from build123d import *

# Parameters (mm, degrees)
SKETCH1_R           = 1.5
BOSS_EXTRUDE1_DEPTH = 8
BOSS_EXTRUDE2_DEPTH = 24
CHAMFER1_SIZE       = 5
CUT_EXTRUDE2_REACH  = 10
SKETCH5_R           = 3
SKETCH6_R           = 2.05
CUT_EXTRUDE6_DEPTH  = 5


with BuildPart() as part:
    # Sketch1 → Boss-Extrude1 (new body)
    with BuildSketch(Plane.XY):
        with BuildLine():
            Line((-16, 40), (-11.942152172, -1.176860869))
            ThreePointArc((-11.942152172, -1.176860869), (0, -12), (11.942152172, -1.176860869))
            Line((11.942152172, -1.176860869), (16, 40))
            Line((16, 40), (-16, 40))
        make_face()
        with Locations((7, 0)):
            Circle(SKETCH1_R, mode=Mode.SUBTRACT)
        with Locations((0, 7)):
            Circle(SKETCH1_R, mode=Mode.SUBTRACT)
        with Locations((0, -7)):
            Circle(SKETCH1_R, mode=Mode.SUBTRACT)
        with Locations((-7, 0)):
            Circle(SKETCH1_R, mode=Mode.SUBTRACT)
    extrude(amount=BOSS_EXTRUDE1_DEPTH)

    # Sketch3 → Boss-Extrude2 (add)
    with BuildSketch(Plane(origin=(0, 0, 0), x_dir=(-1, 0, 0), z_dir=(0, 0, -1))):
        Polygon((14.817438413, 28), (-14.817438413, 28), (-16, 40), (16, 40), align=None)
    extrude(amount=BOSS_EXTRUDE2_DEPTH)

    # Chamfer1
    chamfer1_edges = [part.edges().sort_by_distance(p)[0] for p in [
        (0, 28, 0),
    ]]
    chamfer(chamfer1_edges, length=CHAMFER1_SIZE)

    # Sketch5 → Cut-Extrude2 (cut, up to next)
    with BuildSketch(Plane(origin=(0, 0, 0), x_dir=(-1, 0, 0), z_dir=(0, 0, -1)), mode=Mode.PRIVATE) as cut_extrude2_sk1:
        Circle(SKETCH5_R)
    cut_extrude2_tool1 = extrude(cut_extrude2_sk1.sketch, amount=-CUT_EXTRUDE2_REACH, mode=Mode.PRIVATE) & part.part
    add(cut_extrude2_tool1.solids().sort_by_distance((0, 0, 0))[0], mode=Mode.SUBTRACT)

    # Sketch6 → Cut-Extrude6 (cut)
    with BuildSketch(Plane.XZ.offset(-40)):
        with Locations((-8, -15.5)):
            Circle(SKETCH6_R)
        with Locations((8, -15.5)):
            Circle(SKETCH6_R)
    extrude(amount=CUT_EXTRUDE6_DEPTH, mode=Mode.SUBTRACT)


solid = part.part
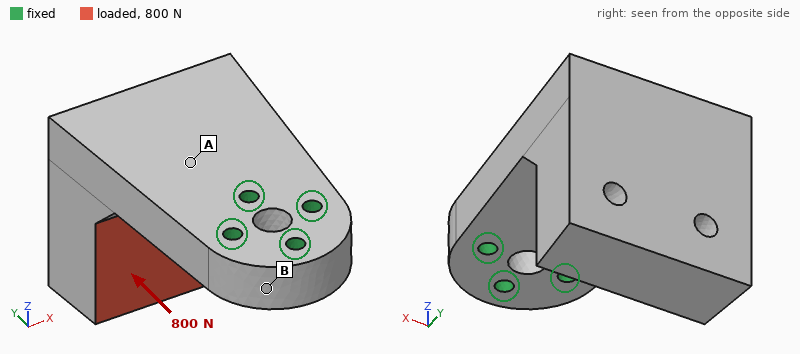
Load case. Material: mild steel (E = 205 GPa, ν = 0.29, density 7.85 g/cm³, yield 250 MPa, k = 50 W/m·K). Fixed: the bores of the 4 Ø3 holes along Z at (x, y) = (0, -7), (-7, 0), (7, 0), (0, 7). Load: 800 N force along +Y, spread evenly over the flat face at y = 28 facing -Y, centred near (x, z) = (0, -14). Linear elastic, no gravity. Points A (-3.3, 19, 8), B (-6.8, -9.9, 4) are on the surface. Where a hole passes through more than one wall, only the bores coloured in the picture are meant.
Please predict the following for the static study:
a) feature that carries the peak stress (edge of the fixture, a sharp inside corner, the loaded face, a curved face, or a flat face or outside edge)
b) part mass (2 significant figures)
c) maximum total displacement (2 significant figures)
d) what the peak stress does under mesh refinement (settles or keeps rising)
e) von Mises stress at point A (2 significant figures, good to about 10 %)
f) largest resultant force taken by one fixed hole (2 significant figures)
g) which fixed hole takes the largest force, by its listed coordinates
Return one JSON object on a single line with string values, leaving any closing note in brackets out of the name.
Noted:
{"feature that carries the peak stress": "edge of the fixture", "part mass": "150 g", "maximum total displacement": "52 µm", "what the peak stress does under mesh refinement": "keeps rising", "von Mises stress at point A": "41 MPa", "largest resultant force taken by one fixed hole": "790 N", "which fixed hole takes the largest force, by its listed coordinates": "(0, 7)"}
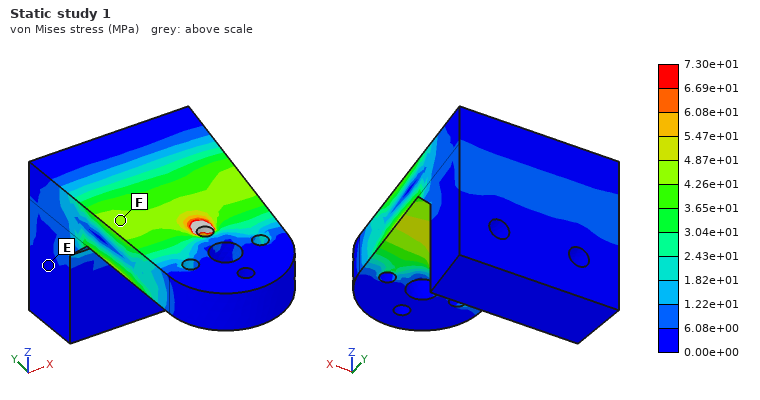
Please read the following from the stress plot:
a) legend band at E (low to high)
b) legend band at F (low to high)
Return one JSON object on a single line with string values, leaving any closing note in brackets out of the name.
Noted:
{"legend band at E": "0.00e+00 to 6.08e+00 MPa", "legend band at F": "4.26e+01 to 4.87e+01 MPa"}
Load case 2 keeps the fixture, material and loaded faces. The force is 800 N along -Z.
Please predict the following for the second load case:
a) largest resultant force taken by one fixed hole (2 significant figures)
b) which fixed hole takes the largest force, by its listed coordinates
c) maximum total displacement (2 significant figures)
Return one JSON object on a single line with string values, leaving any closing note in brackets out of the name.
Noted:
{"largest resultant force taken by one fixed hole": "1.3 kN", "which fixed hole takes the largest force, by its listed coordinates": "(0, 7)", "maximum total displacement": "35 µm"}
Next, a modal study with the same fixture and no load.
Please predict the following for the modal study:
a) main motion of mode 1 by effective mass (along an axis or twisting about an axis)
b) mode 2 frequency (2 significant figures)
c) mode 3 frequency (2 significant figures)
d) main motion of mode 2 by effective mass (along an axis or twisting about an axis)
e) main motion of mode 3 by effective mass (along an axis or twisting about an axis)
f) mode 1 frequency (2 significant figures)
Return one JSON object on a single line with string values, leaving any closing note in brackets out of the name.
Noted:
{"main motion of mode 1 by effective mass": "along Z", "mode 2 frequency": "3500 Hz", "mode 3 frequency": "7500 Hz", "main motion of mode 2 by effective mass": "along X", "main motion of mode 3 by effective mass": "along X", "mode 1 frequency": "2200 Hz"}
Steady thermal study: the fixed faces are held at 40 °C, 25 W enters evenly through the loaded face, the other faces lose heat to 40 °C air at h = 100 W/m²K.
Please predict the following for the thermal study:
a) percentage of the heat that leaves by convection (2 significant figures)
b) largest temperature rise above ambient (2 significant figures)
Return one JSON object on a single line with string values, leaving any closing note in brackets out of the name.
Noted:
{"percentage of the heat that leaves by convection": "50 %", "largest temperature rise above ambient": "48 K"}
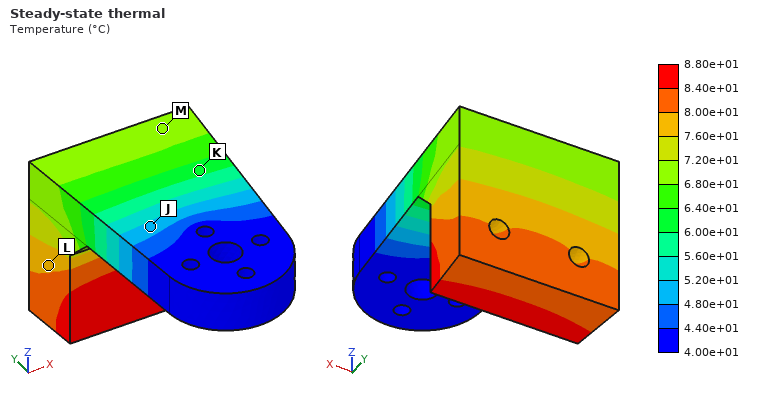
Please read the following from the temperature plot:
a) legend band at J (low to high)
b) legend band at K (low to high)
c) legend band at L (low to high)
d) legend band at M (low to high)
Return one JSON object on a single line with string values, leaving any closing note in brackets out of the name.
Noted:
{"legend band at J": "4.80e+01 to 5.20e+01 °C", "legend band at K": "6.00e+01 to 6.40e+01 °C", "legend band at L": "7.60e+01 to 8.00e+01 °C", "legend band at M": "6.80e+01 to 7.20e+01 °C"}
